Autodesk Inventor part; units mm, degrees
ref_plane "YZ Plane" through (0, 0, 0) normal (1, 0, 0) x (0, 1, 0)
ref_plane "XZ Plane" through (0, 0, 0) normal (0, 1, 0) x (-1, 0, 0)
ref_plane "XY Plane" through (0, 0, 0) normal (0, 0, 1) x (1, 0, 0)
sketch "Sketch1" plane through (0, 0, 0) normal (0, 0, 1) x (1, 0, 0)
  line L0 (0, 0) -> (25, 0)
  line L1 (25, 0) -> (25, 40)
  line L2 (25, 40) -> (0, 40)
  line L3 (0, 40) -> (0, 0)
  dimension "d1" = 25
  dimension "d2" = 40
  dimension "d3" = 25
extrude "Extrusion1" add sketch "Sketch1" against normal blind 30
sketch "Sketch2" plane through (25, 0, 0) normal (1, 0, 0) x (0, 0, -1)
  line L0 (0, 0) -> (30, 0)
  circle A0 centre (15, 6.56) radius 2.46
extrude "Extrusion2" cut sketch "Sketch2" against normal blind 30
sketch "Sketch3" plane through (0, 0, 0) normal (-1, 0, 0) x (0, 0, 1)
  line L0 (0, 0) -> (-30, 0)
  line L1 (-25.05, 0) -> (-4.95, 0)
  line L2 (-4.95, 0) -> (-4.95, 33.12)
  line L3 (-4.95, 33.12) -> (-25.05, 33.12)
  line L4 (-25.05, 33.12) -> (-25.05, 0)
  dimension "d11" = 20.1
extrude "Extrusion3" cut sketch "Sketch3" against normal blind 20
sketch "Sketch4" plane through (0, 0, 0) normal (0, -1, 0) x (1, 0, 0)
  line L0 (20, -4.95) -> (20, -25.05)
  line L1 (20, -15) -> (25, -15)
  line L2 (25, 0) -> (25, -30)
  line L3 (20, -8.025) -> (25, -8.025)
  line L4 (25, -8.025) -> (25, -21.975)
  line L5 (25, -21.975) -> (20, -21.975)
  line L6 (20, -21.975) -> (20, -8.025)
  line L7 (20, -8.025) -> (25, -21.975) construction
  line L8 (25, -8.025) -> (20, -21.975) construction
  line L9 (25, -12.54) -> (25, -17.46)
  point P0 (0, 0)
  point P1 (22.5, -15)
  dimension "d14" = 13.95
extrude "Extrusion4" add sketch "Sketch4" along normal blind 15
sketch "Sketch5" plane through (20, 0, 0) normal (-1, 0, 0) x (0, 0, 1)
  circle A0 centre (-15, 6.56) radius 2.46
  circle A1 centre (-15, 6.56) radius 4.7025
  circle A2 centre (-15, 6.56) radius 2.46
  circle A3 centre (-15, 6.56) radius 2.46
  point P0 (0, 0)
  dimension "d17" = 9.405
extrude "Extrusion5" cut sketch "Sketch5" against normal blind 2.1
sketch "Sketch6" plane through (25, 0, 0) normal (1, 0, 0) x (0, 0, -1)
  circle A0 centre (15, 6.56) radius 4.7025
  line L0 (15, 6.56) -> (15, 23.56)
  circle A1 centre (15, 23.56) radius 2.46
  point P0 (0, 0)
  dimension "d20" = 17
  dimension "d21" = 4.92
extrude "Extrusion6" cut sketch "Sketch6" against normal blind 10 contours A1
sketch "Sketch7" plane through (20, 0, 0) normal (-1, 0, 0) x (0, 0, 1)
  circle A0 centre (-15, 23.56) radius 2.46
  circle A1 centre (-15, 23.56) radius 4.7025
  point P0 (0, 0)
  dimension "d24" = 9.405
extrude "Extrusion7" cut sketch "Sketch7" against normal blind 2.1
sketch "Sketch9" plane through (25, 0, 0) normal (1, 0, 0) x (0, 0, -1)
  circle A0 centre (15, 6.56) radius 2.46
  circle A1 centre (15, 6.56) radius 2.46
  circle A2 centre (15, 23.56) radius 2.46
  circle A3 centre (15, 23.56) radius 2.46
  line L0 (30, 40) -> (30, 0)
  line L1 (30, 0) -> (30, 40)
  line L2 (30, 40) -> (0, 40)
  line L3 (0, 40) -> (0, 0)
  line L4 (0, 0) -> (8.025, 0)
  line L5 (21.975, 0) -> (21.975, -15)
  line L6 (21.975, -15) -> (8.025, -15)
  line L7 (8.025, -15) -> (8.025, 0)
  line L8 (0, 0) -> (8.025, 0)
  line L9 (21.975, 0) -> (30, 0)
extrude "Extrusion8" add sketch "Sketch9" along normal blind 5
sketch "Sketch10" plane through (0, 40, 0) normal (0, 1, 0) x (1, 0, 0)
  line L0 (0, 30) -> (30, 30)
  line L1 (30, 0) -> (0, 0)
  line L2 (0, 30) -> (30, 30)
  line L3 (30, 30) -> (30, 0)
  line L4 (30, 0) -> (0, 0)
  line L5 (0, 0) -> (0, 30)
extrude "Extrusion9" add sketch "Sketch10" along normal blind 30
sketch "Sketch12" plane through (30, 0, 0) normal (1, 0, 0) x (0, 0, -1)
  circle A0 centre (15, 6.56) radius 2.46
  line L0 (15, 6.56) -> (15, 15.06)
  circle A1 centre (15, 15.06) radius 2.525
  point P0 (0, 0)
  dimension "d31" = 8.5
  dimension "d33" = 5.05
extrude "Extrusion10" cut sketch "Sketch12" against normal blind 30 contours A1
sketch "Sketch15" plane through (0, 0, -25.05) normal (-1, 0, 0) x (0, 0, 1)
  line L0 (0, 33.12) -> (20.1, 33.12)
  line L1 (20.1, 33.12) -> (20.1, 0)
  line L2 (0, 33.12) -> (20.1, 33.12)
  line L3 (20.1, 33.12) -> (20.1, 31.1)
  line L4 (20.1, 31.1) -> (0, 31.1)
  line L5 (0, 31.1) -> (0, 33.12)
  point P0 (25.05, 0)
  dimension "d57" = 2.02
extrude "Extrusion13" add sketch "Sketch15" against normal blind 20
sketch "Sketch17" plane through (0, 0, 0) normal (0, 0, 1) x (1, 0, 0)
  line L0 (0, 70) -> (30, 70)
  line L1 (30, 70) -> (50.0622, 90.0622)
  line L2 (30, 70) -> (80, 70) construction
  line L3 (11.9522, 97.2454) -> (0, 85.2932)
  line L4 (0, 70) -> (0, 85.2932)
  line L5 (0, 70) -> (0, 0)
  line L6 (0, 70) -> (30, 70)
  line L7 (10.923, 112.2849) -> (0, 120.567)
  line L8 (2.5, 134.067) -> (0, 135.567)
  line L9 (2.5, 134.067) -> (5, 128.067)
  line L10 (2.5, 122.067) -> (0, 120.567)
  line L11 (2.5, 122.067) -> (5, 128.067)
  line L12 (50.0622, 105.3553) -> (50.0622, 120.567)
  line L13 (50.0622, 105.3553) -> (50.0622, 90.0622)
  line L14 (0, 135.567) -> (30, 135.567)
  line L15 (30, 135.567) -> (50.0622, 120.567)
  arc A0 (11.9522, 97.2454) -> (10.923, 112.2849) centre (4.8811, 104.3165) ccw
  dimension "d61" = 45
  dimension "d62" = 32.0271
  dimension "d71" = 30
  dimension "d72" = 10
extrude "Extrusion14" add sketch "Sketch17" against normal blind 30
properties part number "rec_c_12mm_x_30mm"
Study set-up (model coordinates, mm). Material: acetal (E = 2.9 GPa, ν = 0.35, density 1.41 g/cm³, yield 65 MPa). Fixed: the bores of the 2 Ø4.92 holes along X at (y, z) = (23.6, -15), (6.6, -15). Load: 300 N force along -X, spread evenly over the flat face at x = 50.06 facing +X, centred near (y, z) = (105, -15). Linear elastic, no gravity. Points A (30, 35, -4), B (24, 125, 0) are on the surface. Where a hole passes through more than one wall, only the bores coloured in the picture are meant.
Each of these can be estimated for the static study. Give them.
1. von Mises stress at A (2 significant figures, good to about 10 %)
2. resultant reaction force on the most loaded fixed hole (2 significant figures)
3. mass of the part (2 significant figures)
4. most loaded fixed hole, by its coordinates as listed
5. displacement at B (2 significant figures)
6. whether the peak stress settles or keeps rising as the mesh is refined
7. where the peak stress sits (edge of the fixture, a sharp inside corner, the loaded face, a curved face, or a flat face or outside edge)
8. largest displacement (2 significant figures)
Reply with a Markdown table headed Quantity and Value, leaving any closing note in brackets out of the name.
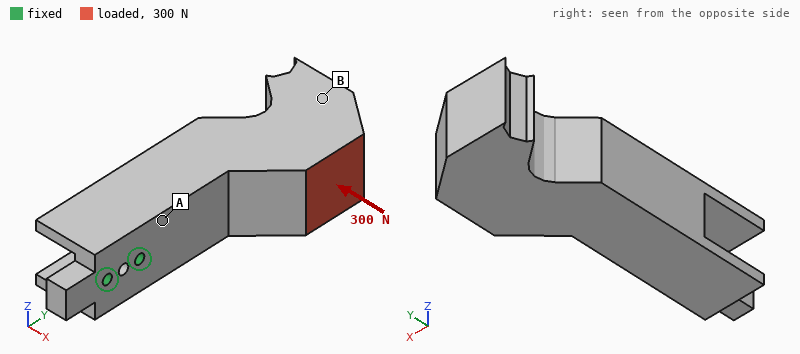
| Quantity | Value |
|---|---|
| von Mises stress at A | 6.1 MPa |
| resultant reaction force on the most loaded fixed hole | 1.3 kN |
| mass of the part | 180 g |
| most loaded fixed hole, by its coordinates as listed | (23.6, -15) |
| displacement at B | 1.6 mm |
| whether the peak stress settles or keeps rising as the mesh is refined | keeps rising |
| where the peak stress sits | edge of the fixture |
| largest displacement | 1.9 mm |
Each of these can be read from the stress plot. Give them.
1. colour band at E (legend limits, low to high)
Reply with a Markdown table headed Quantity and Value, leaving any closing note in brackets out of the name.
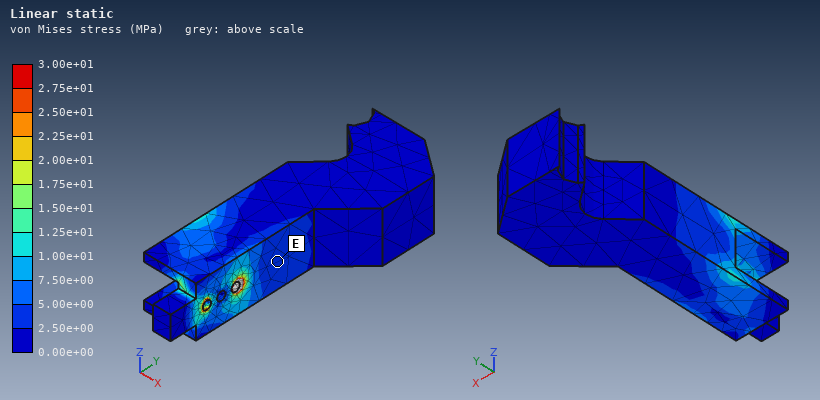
| Quantity | Value |
|---|---|
| colour band at E | 2.50e+00 to 5.00e+00 MPa |
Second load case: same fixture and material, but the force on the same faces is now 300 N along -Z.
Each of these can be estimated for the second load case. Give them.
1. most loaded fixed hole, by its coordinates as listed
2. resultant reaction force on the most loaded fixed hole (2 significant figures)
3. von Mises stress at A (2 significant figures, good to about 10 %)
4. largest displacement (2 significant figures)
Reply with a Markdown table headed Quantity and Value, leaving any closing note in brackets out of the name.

| Quantity | Value |
|---|---|
| most loaded fixed hole, by its coordinates as listed | (23.6, -15) |
| resultant reaction force on the most loaded fixed hole | 1.4 kN |
| von Mises stress at A | 10 MPa |
| largest displacement | 1.7 mm |
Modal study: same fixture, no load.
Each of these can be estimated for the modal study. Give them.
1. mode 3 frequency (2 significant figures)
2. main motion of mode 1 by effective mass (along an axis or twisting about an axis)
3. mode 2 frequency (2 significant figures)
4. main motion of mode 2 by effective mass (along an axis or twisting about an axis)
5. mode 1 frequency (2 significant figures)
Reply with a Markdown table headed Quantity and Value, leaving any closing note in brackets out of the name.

| Quantity | Value |
|---|---|
| mode 3 frequency | 680 Hz |
| main motion of mode 1 by effective mass | along X |
| mode 2 frequency | 260 Hz |
| main motion of mode 2 by effective mass | along Z |
| mode 1 frequency | 220 Hz |
